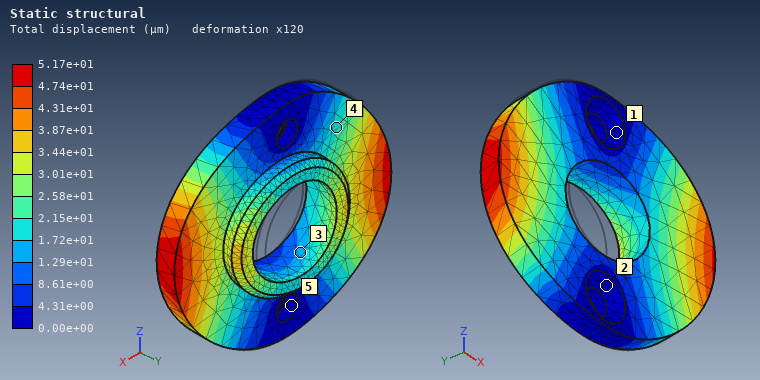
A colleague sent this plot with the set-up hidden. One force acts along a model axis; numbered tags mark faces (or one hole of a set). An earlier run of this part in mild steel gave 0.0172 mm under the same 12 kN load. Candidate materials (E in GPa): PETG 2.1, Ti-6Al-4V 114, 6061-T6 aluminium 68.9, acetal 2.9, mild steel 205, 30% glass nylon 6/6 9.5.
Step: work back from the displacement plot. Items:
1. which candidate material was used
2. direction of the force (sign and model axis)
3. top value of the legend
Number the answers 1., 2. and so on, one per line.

1. 6061-T6 aluminium
2. +X
3. 5.17e+01 µm
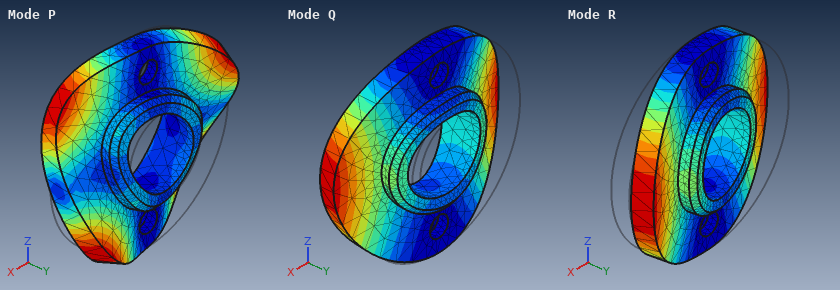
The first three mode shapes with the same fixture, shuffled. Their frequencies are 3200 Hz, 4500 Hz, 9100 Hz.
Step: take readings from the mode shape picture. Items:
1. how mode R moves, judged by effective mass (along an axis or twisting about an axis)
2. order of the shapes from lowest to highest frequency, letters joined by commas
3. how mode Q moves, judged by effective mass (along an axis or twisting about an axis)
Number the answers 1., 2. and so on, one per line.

1. twisting about Z
2. R, Q, P
3. along Y
